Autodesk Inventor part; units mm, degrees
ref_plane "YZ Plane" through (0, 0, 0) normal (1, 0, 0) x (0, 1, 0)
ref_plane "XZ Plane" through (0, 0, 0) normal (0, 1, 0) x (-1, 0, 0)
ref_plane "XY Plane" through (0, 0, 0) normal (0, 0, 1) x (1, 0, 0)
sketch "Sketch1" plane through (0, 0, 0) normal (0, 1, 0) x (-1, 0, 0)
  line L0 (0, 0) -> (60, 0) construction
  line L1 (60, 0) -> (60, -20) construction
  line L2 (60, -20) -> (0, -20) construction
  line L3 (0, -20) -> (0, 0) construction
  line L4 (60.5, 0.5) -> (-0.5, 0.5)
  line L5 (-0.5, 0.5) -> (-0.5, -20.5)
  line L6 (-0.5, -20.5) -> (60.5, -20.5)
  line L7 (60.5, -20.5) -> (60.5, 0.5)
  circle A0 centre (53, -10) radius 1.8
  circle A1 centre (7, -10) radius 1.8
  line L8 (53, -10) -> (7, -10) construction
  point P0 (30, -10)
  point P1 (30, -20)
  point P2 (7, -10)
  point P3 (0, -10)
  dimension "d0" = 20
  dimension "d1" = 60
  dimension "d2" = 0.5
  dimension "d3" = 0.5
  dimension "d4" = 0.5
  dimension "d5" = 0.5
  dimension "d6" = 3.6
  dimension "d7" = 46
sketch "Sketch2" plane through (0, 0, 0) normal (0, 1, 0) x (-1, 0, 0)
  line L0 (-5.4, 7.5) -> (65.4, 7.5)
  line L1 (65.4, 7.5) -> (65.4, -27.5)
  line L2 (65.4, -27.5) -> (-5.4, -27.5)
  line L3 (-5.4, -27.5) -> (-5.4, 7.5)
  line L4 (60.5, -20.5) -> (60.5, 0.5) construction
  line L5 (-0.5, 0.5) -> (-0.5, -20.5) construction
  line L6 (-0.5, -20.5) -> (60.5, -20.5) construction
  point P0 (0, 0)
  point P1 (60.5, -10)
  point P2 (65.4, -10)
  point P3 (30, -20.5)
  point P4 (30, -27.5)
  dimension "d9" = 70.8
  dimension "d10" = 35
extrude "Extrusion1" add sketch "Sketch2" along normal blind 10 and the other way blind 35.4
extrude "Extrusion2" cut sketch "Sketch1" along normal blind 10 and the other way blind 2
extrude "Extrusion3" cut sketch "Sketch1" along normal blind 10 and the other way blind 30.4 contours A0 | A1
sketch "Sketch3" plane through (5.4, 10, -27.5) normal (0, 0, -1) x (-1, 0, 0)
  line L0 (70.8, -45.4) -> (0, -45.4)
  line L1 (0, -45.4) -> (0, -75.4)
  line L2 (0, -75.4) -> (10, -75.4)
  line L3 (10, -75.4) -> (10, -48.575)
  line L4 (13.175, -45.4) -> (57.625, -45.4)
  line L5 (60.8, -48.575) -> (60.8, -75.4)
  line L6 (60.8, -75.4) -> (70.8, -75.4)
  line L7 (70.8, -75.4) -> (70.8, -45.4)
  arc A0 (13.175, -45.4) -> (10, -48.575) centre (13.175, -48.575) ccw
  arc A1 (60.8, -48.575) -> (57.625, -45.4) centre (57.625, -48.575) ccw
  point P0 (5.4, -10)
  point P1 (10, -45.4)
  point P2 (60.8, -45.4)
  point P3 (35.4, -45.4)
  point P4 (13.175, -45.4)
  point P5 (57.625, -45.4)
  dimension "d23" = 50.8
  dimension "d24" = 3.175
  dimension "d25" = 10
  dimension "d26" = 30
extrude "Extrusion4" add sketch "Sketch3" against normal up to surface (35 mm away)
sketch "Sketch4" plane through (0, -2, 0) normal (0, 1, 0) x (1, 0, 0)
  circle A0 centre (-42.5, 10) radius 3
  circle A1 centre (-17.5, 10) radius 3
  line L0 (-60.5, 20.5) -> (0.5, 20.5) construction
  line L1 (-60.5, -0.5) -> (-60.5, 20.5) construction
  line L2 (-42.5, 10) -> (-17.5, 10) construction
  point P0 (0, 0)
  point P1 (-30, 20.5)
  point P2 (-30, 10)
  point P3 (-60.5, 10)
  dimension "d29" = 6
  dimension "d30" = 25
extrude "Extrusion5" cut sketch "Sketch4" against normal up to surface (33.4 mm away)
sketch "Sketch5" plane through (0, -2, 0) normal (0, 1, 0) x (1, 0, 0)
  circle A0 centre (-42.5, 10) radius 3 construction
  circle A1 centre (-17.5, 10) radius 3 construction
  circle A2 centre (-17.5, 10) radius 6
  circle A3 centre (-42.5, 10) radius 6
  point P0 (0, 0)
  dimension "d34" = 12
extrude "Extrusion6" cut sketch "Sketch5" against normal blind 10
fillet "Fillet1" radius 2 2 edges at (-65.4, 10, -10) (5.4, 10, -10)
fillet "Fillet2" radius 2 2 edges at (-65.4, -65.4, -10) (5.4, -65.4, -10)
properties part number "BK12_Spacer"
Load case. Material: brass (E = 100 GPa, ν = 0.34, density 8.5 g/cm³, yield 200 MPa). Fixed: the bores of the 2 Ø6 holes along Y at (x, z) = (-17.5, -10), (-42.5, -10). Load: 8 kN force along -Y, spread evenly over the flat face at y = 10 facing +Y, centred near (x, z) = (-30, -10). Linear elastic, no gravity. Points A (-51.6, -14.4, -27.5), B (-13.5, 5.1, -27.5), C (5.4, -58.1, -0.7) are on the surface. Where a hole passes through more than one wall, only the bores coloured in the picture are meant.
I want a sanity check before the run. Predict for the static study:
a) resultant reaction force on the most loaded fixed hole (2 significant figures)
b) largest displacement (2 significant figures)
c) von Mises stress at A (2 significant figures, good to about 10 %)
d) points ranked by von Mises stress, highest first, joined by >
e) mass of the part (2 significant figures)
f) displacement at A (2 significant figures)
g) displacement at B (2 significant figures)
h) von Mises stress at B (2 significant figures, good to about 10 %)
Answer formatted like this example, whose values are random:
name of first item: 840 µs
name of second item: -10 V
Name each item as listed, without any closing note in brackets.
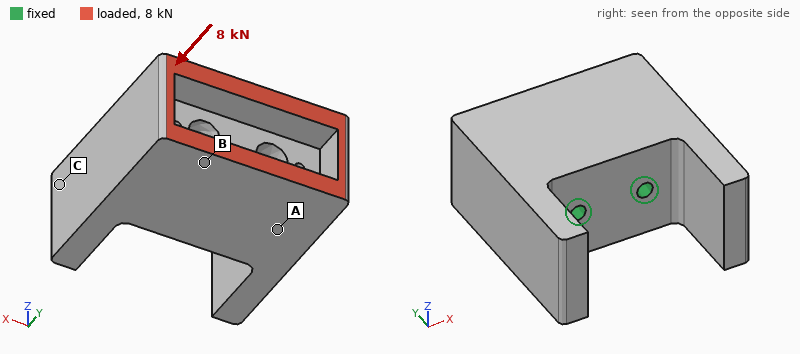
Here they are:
resultant reaction force on the most loaded fixed hole: 4.0 kN
largest displacement: 4.1 µm
von Mises stress at A: 4.7 MPa
points ranked by von Mises stress, highest first, joined by >: B > A > C
mass of the part: 970 g
displacement at A: 2.0 µm
displacement at B: 3.6 µm
von Mises stress at B: 8.5 MPa
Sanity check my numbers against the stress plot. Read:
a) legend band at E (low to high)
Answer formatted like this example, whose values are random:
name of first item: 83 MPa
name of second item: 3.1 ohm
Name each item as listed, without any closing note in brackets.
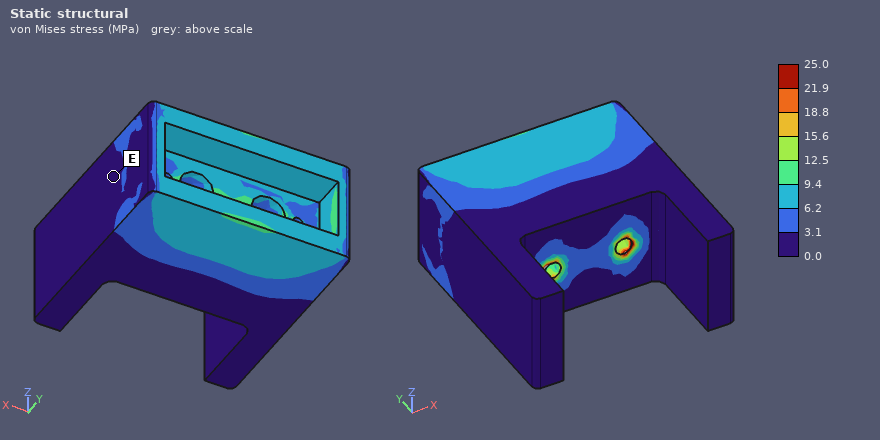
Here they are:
legend band at E: 0.0 to 3.1 MPa
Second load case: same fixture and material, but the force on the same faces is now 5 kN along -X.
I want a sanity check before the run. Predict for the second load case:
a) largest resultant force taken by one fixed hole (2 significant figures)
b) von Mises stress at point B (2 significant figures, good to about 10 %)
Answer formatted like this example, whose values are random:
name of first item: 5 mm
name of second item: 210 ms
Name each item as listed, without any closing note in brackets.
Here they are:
largest resultant force taken by one fixed hole: 4.3 kN
von Mises stress at point B: 10 MPa
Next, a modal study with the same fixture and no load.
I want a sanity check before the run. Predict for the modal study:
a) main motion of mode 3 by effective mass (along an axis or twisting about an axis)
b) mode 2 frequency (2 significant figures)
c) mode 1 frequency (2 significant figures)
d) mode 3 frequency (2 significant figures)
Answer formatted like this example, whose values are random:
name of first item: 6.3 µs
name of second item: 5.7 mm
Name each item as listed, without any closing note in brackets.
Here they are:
main motion of mode 3 by effective mass: twisting about X
mode 2 frequency: 4300 Hz
mode 1 frequency: 4200 Hz
mode 3 frequency: 5200 Hz
